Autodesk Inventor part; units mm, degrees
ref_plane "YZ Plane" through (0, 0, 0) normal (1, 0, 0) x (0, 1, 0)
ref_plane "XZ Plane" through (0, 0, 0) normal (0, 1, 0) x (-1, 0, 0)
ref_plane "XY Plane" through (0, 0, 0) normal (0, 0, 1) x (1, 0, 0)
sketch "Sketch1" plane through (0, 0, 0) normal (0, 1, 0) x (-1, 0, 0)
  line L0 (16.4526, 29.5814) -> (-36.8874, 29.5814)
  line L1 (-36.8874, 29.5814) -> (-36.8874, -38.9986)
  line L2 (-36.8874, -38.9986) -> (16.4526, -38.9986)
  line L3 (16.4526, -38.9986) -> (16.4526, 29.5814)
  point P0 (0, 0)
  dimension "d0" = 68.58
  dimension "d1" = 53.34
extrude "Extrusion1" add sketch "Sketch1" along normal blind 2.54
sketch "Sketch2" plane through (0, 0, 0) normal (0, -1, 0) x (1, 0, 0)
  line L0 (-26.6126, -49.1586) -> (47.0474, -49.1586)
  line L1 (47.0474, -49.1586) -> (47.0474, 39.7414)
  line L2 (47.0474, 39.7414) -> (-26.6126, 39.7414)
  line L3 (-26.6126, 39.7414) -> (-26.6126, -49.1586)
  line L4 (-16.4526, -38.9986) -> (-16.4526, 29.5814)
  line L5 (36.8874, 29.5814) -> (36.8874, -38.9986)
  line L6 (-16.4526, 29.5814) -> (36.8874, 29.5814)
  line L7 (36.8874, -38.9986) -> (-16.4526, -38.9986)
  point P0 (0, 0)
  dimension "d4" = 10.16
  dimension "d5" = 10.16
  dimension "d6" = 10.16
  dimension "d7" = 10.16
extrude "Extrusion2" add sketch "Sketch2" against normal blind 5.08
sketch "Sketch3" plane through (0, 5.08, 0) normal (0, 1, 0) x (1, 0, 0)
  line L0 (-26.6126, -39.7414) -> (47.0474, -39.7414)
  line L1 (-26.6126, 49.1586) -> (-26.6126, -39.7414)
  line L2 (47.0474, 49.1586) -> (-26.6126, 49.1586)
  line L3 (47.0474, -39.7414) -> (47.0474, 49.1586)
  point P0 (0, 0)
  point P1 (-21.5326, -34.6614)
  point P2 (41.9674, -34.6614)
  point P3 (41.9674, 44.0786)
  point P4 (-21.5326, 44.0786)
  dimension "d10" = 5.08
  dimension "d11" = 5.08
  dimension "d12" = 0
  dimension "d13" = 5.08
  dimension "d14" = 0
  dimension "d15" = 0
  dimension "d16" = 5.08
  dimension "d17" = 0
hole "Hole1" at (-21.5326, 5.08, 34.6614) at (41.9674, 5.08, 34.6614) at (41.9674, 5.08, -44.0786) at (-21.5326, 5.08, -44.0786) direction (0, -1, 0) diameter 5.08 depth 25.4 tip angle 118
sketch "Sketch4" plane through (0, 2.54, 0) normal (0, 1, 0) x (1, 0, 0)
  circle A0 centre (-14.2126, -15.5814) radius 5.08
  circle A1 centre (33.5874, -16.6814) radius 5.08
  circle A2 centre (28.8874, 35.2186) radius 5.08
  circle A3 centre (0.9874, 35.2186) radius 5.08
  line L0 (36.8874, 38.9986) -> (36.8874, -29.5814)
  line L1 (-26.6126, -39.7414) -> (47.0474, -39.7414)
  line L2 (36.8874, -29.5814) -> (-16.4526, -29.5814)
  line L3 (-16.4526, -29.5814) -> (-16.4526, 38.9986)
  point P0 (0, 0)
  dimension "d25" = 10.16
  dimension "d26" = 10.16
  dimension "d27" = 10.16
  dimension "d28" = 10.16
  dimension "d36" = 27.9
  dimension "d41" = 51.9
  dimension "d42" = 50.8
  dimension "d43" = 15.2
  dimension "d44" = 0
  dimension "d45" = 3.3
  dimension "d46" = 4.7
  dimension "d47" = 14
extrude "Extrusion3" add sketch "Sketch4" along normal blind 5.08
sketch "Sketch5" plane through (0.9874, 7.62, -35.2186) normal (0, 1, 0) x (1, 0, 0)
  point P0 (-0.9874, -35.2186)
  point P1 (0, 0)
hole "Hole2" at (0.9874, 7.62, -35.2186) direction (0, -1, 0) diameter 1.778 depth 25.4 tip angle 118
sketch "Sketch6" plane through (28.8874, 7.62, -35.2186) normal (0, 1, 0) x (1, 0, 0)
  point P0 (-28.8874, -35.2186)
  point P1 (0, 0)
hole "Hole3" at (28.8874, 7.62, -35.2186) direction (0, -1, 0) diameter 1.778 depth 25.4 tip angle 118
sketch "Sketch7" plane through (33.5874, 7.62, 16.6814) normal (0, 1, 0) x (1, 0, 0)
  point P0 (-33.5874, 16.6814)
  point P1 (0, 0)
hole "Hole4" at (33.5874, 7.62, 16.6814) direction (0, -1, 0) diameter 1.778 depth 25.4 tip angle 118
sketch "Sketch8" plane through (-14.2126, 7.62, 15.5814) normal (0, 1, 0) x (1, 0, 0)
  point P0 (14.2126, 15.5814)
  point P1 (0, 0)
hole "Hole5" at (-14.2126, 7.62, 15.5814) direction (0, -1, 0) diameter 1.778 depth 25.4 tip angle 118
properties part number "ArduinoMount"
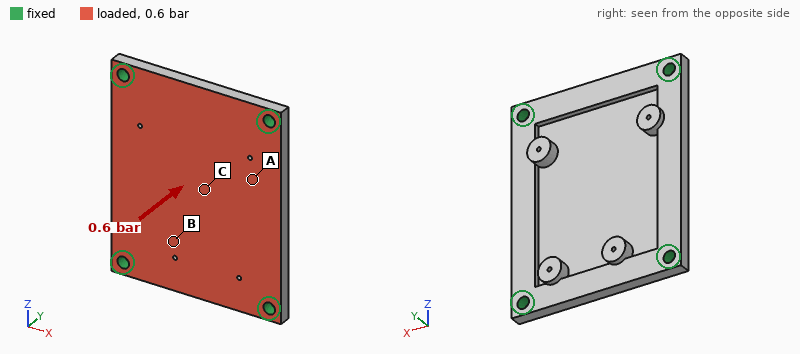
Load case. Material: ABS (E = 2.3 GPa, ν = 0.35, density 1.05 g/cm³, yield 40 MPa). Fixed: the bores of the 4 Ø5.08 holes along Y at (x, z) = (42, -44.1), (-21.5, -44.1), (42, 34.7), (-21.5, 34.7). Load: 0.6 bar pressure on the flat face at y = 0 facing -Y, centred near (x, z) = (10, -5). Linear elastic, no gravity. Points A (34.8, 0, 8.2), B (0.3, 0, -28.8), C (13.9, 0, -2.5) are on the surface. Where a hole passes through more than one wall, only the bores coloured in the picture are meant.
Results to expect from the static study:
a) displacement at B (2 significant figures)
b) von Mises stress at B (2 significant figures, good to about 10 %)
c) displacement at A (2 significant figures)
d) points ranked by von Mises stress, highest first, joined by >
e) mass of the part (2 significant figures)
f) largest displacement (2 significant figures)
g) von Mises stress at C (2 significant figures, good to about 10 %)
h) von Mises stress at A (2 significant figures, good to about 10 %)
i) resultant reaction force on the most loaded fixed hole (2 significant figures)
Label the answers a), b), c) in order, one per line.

a) 0.48 mm
b) 2.3 MPa
c) 0.48 mm
d) C > A > B
e) 26 g
f) 0.96 mm
g) 8.5 MPa
h) 4.2 MPa
i) 130 N
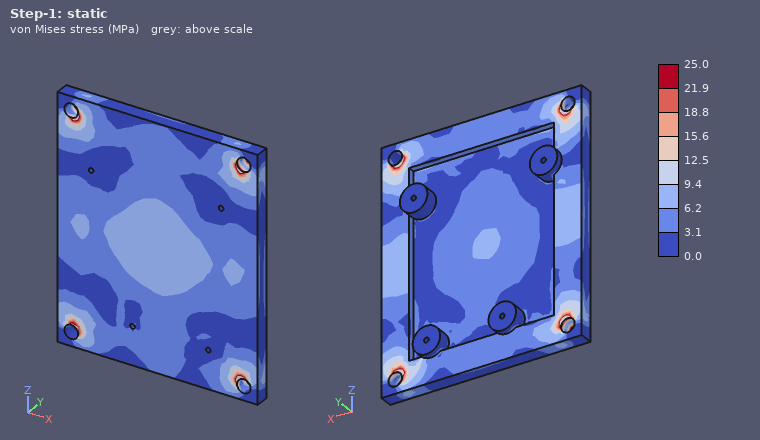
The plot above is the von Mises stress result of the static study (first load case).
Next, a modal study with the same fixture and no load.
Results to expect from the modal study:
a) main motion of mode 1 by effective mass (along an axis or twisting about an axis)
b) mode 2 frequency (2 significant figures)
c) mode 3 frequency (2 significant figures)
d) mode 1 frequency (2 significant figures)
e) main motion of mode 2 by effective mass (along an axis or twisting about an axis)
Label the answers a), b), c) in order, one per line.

a) along Y
b) 1300 Hz
c) 1600 Hz
d) 910 Hz
e) twisting about Z
